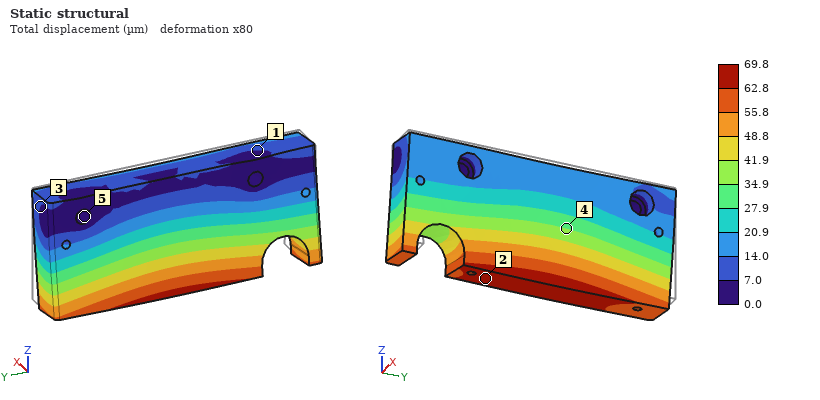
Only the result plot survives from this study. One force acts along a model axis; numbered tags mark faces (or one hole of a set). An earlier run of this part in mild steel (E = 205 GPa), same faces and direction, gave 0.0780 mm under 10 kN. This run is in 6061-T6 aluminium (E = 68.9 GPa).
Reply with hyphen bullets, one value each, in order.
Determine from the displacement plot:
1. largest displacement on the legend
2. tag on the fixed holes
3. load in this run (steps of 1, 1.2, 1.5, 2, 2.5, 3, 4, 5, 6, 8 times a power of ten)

- 69.8 µm
- 5
- 3 kN
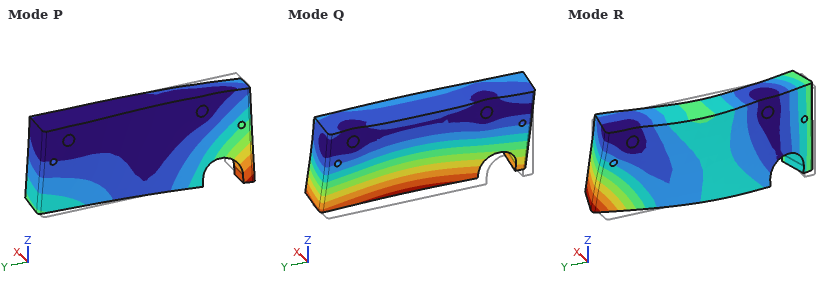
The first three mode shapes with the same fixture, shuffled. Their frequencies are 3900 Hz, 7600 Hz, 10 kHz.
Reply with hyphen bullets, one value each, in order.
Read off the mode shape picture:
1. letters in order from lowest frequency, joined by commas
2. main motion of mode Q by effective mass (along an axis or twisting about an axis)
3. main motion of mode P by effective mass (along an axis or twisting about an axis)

- Q, P, R
- along X
- twisting about Z
